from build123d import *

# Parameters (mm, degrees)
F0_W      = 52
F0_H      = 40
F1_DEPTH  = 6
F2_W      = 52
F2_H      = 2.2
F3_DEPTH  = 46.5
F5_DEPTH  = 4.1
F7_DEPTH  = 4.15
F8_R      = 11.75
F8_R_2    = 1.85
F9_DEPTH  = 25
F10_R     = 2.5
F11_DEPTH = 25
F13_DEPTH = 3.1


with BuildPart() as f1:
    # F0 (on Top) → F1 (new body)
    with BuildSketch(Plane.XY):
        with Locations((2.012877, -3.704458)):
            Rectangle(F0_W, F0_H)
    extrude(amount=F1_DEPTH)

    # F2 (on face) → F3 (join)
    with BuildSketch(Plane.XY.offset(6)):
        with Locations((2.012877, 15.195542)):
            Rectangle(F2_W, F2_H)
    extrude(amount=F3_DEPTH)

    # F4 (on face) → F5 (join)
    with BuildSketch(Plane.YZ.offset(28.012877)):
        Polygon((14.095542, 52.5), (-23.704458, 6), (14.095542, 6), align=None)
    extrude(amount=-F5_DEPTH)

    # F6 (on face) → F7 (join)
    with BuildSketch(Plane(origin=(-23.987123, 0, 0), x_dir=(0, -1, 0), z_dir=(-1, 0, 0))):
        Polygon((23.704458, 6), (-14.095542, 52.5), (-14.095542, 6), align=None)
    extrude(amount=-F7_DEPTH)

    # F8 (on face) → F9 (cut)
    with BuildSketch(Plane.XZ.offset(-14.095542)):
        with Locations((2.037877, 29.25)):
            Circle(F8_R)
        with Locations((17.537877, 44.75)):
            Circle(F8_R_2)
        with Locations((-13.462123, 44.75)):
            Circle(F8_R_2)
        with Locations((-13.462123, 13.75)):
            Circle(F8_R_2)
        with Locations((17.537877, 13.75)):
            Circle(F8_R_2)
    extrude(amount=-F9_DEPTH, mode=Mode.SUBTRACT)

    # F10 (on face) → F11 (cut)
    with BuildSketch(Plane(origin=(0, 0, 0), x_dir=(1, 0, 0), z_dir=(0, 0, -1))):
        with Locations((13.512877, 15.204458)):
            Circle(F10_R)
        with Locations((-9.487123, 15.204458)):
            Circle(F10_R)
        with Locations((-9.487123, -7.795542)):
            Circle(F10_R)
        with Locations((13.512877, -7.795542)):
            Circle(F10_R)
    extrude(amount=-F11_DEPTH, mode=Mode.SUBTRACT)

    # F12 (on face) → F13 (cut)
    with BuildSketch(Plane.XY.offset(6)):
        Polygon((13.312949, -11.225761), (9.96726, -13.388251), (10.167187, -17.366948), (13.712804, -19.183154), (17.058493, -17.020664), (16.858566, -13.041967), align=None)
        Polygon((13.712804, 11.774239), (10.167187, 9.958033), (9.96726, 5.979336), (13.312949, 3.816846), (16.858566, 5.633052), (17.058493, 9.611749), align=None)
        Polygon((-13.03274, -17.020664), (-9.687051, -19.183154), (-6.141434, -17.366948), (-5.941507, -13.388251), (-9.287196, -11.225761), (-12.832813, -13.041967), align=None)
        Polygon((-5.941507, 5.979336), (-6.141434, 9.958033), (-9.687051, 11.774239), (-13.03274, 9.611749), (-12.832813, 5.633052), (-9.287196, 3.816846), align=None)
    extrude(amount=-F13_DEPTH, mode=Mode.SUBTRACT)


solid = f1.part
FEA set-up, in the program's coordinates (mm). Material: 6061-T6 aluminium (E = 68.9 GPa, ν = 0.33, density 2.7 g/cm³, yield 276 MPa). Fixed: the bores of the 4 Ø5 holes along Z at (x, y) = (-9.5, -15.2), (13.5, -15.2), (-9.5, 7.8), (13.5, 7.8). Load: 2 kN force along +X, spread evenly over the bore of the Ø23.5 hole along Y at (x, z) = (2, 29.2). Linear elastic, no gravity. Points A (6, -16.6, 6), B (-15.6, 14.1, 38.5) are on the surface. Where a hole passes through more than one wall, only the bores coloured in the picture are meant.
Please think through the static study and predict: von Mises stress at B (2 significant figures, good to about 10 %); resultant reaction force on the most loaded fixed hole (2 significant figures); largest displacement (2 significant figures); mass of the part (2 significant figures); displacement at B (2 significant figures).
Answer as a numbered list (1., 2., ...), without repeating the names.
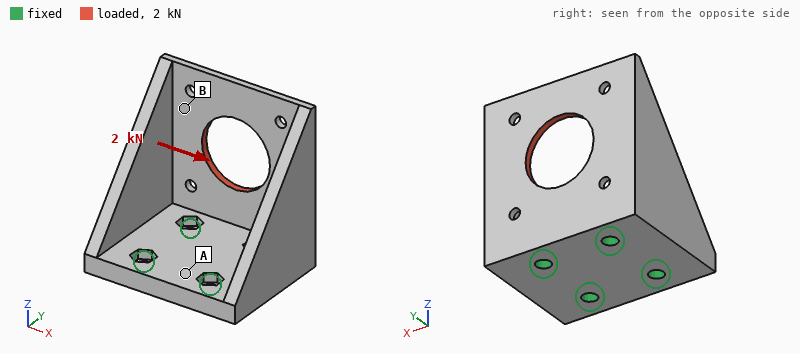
1. 31 MPa
2. 2.3 kN
3. 0.16 mm
4. 63 g
5. 0.12 mm
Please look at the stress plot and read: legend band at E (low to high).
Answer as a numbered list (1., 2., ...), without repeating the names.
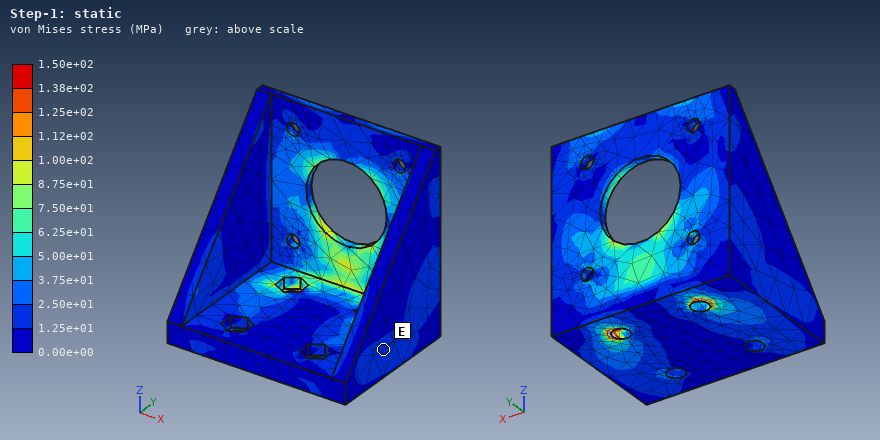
1. 1.25e+01 to 2.50e+01 MPa
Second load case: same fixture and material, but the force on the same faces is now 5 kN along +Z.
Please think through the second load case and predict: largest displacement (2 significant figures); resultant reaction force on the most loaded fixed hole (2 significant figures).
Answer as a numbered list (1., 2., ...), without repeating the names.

1. 0.12 mm
2. 3.1 kN
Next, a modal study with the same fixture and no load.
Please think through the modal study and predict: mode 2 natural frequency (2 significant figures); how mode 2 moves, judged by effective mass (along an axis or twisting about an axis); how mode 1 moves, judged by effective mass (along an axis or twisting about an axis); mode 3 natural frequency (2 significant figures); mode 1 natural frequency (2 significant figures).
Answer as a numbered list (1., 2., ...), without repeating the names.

1. 4000 Hz
2. along X
3. along Y
4. 5900 Hz
5. 3800 Hz
